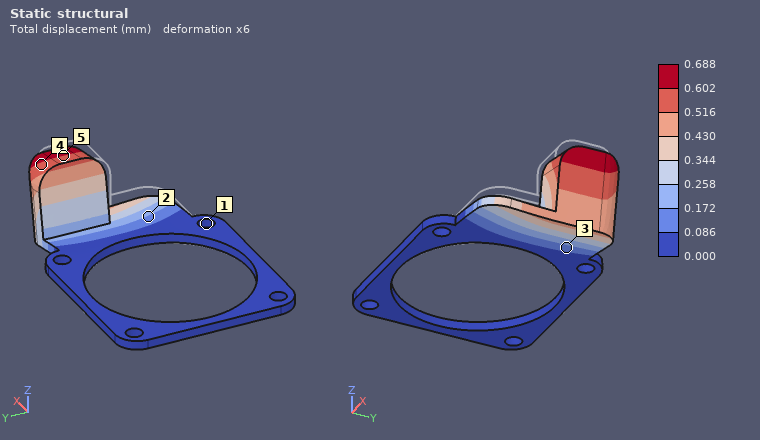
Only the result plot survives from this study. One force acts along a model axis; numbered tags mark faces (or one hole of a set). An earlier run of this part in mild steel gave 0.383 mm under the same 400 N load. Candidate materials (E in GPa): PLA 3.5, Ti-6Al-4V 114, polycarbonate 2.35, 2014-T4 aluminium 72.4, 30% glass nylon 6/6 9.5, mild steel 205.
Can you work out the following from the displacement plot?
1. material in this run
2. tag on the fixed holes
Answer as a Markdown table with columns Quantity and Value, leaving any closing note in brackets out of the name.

| Quantity | Value |
|---|---|
| material in this run | Ti-6Al-4V |
| tag on the fixed holes | 1 |
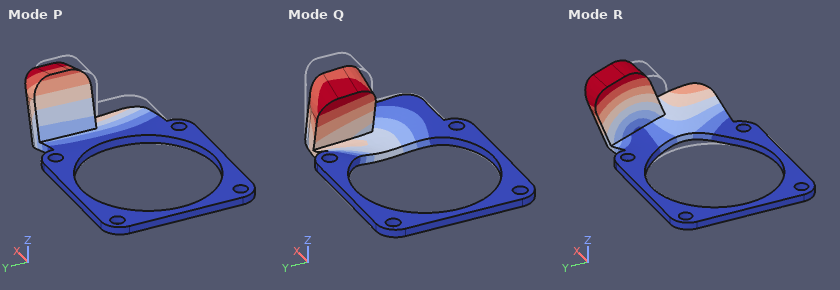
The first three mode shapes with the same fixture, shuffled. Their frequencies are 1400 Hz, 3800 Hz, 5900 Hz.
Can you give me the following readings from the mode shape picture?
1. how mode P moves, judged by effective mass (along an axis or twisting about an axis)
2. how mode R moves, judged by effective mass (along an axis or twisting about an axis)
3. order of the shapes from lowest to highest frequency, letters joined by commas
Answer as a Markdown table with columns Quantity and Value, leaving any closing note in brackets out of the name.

| Quantity | Value |
|---|---|
| how mode P moves, judged by effective mass | along Z |
| how mode R moves, judged by effective mass | along Y |
| order of the shapes from lowest to highest frequency, letters joined by commas | P, R, Q |
